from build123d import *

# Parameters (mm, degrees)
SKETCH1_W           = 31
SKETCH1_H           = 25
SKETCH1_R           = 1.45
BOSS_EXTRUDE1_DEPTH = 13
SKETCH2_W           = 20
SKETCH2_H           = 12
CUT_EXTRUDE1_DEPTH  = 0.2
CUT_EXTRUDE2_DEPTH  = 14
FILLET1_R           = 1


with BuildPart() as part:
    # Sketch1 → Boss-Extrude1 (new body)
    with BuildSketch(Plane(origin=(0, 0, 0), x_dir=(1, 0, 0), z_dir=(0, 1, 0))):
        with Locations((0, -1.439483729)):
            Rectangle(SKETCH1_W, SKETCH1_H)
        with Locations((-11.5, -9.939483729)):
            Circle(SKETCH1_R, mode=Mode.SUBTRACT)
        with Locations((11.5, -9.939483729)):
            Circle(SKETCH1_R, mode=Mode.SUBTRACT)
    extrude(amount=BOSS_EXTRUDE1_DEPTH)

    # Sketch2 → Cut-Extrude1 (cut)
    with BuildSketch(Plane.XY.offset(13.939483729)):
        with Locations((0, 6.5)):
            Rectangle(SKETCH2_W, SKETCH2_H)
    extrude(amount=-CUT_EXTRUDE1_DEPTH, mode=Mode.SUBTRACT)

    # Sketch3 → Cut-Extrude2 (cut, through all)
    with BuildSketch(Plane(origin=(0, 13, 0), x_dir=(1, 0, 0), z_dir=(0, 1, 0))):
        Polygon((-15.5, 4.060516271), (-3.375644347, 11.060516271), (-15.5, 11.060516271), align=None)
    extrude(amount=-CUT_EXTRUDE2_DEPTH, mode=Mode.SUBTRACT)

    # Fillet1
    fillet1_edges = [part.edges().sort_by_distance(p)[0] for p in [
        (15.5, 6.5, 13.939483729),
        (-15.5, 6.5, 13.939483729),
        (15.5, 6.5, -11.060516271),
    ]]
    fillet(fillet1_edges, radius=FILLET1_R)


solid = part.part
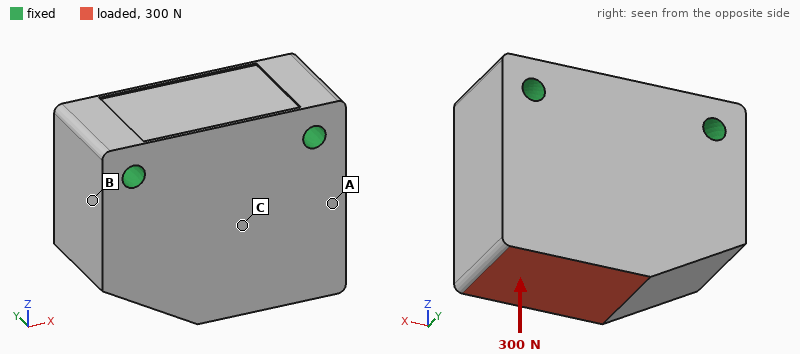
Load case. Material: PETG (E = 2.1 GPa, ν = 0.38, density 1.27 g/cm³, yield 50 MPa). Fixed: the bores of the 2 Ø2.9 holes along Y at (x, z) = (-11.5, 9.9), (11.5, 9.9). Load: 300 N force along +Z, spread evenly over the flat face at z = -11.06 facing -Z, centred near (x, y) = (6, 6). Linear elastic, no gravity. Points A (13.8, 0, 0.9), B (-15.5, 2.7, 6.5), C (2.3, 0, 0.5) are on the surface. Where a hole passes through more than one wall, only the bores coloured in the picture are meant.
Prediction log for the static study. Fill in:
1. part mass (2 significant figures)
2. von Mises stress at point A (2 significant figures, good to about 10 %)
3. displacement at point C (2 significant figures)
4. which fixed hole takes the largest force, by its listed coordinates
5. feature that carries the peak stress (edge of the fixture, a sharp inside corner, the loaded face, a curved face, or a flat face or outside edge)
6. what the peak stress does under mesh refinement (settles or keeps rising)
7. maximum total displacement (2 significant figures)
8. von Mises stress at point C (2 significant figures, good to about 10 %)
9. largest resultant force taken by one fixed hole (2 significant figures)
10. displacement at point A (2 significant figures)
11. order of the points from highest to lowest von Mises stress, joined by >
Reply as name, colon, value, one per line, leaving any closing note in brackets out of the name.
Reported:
part mass: 12 g
von Mises stress at point A: 1.4 MPa
displacement at point C: 7.8 µm
which fixed hole takes the largest force, by its listed coordinates: (11.5, 9.9)
feature that carries the peak stress: edge of the fixture
what the peak stress does under mesh refinement: keeps rising
maximum total displacement: 16 µm
von Mises stress at point C: 0.74 MPa
largest resultant force taken by one fixed hole: 220 N
displacement at point A: 8.2 µm
order of the points from highest to lowest von Mises stress, joined by >: A > C > B
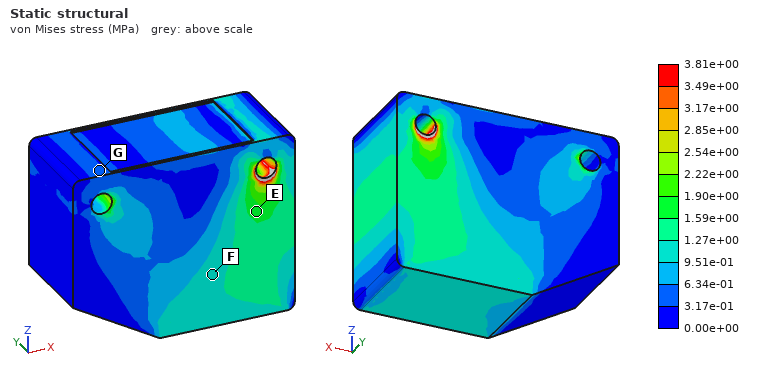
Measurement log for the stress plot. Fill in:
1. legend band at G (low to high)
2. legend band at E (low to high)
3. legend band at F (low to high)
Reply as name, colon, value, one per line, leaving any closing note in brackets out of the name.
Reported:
legend band at G: 3.17e-01 to 6.34e-01 MPa
legend band at E: 1.59e+00 to 1.90e+00 MPa
legend band at F: 9.51e-01 to 1.27e+00 MPa
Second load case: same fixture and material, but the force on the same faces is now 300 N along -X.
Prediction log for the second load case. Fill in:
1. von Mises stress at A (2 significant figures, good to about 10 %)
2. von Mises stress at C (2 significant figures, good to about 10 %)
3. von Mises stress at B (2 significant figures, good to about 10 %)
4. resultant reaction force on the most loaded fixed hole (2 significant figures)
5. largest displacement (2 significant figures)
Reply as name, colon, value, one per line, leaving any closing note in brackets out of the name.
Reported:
von Mises stress at A: 1.8 MPa
von Mises stress at C: 1.7 MPa
von Mises stress at B: 1.7 MPa
resultant reaction force on the most loaded fixed hole: 310 N
largest displacement: 54 µm
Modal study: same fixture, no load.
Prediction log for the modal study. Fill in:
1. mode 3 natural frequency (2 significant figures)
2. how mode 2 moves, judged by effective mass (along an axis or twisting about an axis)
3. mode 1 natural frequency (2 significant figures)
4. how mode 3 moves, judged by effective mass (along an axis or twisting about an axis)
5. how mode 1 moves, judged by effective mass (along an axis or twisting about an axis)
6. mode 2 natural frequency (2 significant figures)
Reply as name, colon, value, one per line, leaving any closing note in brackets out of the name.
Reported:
mode 3 natural frequency: 8100 Hz
how mode 2 moves, judged by effective mass: along X
mode 1 natural frequency: 4200 Hz
how mode 3 moves, judged by effective mass: twisting about Z
how mode 1 moves, judged by effective mass: along Y
mode 2 natural frequency: 7500 Hz
